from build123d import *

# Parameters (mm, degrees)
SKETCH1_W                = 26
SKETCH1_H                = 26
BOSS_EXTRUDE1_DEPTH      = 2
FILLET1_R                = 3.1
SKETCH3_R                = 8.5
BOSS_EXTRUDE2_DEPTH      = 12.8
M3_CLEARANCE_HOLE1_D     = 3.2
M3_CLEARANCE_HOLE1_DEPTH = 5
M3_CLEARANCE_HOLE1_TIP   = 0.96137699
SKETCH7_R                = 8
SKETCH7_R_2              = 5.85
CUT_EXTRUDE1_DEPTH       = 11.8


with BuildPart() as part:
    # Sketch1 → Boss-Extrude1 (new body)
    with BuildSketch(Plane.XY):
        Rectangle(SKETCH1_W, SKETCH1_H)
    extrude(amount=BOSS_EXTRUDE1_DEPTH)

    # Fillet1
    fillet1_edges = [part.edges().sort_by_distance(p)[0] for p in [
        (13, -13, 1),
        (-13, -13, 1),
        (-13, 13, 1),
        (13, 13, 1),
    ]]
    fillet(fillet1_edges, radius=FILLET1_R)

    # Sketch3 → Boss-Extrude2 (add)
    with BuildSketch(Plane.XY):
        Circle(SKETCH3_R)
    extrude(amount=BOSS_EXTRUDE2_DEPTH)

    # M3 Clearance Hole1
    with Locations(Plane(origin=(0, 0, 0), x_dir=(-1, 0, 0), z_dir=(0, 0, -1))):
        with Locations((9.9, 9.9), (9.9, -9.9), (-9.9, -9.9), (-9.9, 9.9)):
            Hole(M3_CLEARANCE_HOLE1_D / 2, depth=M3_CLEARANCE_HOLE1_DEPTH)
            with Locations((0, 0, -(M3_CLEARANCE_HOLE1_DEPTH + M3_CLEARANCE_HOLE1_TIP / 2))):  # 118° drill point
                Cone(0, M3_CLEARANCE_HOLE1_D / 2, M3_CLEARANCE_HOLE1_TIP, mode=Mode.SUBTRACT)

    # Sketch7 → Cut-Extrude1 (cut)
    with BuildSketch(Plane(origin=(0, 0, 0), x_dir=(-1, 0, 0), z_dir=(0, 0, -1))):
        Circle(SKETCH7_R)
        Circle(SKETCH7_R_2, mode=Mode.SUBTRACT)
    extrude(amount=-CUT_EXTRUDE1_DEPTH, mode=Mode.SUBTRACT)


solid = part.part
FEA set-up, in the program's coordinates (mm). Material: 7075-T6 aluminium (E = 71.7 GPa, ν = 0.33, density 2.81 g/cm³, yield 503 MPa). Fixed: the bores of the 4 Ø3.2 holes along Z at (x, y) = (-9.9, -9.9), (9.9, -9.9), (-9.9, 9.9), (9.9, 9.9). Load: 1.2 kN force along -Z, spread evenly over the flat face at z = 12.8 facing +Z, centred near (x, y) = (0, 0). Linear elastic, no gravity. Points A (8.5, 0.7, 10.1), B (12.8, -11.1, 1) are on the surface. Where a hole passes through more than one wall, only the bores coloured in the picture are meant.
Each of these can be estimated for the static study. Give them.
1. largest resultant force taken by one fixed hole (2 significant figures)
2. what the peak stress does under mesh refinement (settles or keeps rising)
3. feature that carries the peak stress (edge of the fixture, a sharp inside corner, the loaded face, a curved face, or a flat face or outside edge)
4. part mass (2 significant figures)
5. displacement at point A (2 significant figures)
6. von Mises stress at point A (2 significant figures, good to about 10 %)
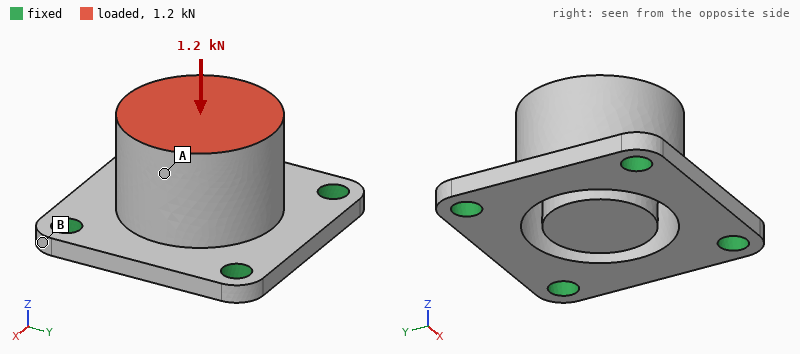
310 N
keeps rising
edge of the fixture
7.4 g
30 µm
52 MPa
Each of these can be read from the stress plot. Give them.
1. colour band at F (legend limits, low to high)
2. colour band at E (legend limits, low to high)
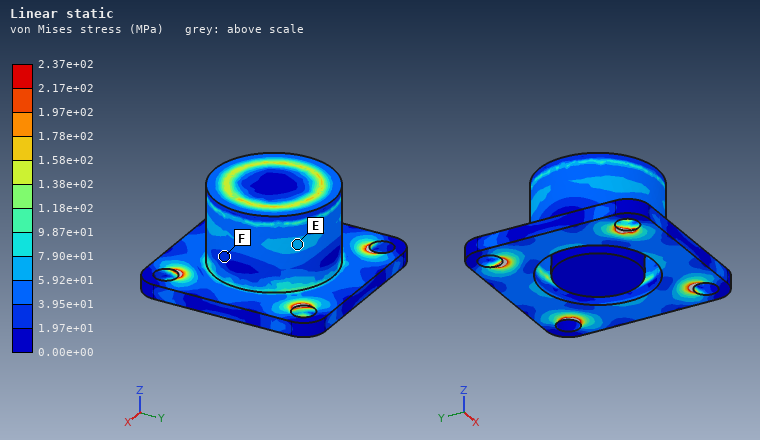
1.97e+01 to 3.95e+01 MPa
5.92e+01 to 7.90e+01 MPa
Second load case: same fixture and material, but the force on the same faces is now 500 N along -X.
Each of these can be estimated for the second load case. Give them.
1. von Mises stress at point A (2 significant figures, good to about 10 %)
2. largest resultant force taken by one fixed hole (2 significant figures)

22 MPa
230 N
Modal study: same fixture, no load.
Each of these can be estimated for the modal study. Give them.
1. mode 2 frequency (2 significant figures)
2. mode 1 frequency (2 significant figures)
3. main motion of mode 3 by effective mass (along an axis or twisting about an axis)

8500 Hz
8500 Hz
along Z
